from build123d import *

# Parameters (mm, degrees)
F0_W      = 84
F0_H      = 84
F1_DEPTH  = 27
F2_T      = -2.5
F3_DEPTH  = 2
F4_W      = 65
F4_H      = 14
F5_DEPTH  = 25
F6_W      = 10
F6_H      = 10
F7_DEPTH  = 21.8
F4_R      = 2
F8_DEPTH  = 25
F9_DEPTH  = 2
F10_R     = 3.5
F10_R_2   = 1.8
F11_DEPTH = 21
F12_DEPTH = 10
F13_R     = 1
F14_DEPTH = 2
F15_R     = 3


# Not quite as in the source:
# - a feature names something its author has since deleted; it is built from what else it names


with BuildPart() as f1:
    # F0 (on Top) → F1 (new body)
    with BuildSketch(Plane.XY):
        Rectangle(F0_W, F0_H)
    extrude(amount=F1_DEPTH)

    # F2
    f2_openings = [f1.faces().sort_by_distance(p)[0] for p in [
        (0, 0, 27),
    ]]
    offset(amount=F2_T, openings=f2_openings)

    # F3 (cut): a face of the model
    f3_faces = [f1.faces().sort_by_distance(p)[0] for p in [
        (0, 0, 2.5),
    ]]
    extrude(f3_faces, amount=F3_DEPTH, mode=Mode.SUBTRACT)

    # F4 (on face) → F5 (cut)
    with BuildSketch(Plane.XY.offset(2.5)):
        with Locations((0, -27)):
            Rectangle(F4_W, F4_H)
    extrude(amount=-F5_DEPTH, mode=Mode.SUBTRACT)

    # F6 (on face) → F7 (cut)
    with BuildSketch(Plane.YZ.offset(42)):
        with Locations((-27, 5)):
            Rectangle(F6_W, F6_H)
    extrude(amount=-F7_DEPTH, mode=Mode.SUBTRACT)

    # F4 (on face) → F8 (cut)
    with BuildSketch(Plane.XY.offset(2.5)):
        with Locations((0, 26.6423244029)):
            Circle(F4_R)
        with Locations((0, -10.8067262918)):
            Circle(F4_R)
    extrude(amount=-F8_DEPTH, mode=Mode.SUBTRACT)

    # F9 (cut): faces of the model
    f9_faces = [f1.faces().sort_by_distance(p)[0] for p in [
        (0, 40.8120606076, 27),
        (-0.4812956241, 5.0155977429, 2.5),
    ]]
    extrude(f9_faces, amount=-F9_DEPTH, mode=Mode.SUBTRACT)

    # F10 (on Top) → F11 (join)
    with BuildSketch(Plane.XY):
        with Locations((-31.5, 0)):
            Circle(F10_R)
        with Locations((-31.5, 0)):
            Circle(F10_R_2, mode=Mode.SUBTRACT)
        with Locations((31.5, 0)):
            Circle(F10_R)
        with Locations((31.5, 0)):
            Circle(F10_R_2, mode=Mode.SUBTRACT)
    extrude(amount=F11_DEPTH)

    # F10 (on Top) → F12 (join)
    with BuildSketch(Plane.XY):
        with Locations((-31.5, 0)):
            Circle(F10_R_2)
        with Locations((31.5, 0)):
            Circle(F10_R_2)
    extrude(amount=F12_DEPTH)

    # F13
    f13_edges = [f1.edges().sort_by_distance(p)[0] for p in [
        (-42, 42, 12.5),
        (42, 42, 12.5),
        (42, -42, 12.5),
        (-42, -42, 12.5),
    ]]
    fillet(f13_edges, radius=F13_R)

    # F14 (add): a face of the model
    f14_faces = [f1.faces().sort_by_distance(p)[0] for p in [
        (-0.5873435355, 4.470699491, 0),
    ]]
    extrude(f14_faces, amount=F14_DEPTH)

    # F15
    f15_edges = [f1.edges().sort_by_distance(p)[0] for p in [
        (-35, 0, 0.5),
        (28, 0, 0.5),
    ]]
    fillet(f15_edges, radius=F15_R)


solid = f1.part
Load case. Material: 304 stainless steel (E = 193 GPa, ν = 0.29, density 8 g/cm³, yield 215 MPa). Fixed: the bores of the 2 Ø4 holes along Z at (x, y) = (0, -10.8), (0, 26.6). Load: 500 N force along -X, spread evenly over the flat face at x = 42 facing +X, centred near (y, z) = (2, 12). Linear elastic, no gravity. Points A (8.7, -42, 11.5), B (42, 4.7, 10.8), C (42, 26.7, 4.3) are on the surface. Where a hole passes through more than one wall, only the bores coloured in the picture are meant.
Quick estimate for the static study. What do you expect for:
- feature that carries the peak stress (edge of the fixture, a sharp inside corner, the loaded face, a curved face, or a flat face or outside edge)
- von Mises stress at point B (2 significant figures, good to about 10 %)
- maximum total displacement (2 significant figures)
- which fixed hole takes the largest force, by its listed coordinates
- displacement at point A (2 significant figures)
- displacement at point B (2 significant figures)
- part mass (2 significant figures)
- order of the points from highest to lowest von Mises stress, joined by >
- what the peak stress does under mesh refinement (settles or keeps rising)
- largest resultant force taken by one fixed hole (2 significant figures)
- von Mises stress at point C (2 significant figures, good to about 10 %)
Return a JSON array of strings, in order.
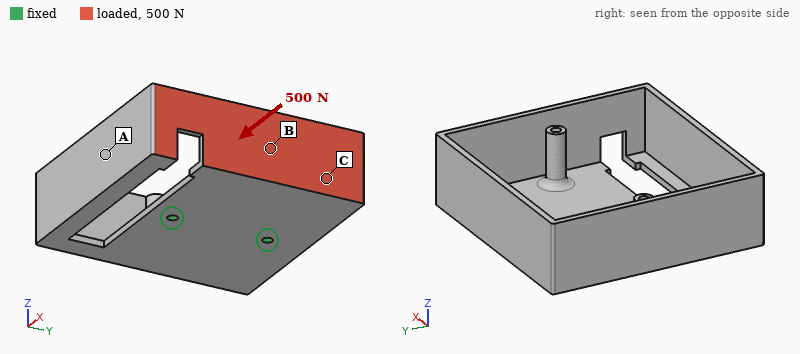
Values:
["edge of the fixture", "17 MPa", "0.21 mm", "(0, -10.8)", "0.080 mm", "0.15 mm", "290 g", "C > B > A", "keeps rising", "340 N", "34 MPa"]
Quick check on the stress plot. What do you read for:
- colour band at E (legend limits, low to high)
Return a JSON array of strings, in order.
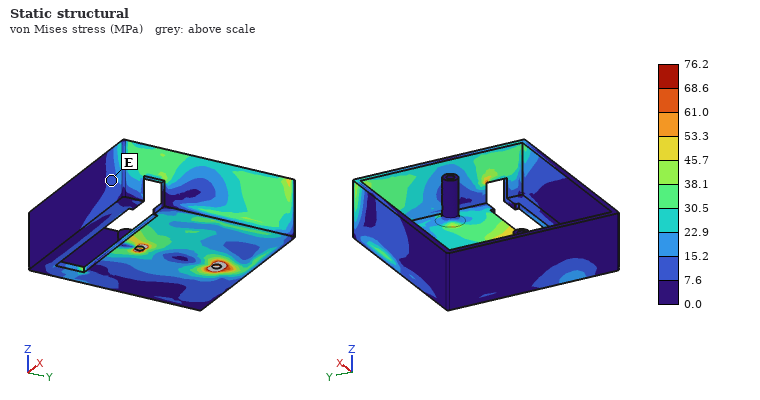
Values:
["7.6 to 15.2 MPa"]
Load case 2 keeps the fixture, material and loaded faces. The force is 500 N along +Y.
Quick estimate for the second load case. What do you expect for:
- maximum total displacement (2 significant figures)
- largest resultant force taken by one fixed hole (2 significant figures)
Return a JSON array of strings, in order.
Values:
["0.18 mm", "610 N"]
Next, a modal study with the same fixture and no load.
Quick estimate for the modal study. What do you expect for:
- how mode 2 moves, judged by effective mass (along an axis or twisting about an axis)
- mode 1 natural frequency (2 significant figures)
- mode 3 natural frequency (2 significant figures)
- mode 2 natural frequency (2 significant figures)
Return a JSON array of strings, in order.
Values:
["along Z", "470 Hz", "880 Hz", "500 Hz"]
